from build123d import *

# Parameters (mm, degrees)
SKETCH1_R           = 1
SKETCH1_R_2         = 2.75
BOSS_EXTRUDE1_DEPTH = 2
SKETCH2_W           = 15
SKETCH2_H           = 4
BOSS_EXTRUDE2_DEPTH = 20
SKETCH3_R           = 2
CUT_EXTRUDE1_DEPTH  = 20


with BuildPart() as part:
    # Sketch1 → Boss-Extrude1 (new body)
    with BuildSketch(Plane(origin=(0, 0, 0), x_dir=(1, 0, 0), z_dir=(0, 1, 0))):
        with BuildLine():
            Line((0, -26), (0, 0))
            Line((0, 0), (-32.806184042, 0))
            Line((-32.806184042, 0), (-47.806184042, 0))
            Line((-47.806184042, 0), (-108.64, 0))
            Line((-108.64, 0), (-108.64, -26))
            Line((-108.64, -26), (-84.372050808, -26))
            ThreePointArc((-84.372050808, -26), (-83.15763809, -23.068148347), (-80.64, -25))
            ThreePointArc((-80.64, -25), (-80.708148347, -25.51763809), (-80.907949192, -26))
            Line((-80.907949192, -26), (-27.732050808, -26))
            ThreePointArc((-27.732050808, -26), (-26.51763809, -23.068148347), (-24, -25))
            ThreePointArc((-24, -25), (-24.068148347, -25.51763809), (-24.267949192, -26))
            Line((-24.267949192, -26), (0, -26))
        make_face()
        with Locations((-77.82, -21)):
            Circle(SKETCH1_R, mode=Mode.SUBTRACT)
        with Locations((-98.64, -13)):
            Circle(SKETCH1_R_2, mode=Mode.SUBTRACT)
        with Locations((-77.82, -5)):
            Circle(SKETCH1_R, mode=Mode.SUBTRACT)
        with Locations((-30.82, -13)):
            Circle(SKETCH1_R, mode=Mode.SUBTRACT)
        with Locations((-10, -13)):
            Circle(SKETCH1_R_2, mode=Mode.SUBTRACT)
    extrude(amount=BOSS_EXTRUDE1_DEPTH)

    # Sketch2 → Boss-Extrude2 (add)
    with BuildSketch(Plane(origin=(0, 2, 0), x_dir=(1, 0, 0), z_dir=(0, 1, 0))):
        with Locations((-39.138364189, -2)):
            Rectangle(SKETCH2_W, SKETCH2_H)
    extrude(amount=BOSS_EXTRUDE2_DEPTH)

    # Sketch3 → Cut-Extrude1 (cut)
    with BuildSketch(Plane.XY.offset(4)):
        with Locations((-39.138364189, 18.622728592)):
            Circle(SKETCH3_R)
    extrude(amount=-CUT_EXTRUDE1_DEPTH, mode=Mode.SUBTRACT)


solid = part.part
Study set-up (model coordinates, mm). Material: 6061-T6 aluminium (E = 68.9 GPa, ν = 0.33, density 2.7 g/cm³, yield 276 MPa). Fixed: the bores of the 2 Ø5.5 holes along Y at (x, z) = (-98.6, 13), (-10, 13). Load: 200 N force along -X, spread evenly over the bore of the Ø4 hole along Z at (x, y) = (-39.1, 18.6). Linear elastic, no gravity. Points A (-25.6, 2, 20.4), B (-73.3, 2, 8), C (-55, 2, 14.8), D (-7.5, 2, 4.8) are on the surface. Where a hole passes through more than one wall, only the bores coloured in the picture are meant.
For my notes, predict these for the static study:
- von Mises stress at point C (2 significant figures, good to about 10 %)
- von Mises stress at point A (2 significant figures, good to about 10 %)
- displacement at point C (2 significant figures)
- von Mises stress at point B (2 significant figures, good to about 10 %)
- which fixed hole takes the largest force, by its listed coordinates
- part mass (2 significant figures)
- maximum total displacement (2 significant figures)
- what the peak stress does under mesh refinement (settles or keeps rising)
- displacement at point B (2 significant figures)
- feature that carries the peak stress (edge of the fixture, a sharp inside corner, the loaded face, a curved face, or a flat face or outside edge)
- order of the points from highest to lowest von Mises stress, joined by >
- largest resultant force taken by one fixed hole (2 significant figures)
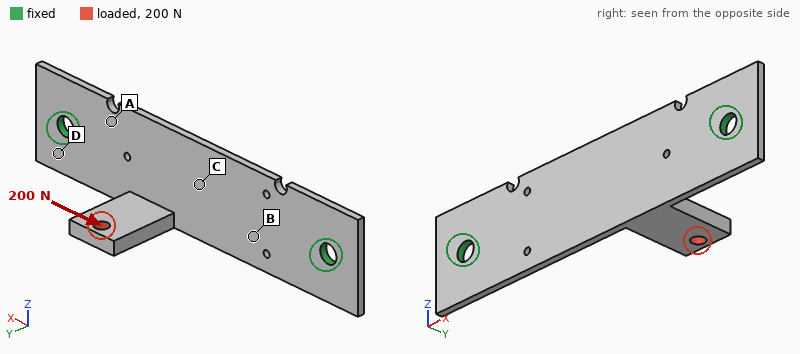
59 MPa
40 MPa
0.27 mm
23 MPa
(-10, 13)
18 g
0.51 mm
keeps rising
0.20 mm
a sharp inside corner
C > A > B > D
140 N
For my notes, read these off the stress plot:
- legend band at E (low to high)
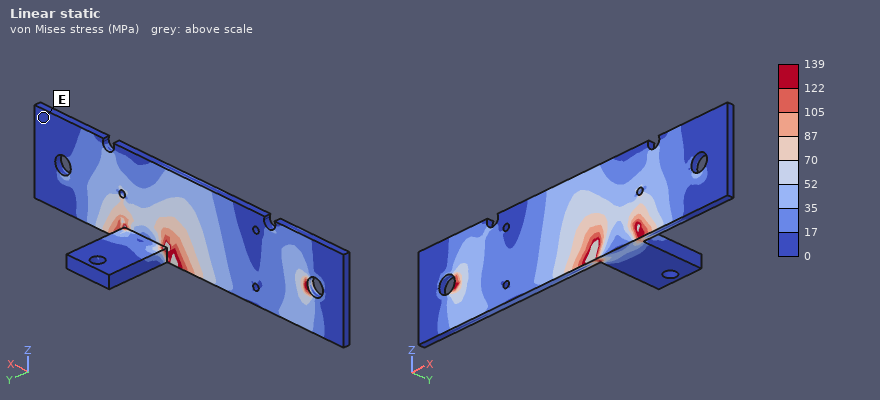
0 to 17 MPa
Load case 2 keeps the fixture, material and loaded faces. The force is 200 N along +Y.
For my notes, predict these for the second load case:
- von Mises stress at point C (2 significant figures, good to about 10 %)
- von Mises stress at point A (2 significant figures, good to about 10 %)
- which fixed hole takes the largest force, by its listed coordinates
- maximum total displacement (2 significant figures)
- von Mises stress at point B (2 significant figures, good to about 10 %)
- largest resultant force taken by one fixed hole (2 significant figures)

59 MPa
60 MPa
(-10, 13)
0.75 mm
40 MPa
150 N
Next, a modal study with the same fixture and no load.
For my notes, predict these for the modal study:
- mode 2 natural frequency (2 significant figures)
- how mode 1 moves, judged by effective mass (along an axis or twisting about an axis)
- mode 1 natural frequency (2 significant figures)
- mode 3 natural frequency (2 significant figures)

1700 Hz
along Y
1100 Hz
3300 Hz
